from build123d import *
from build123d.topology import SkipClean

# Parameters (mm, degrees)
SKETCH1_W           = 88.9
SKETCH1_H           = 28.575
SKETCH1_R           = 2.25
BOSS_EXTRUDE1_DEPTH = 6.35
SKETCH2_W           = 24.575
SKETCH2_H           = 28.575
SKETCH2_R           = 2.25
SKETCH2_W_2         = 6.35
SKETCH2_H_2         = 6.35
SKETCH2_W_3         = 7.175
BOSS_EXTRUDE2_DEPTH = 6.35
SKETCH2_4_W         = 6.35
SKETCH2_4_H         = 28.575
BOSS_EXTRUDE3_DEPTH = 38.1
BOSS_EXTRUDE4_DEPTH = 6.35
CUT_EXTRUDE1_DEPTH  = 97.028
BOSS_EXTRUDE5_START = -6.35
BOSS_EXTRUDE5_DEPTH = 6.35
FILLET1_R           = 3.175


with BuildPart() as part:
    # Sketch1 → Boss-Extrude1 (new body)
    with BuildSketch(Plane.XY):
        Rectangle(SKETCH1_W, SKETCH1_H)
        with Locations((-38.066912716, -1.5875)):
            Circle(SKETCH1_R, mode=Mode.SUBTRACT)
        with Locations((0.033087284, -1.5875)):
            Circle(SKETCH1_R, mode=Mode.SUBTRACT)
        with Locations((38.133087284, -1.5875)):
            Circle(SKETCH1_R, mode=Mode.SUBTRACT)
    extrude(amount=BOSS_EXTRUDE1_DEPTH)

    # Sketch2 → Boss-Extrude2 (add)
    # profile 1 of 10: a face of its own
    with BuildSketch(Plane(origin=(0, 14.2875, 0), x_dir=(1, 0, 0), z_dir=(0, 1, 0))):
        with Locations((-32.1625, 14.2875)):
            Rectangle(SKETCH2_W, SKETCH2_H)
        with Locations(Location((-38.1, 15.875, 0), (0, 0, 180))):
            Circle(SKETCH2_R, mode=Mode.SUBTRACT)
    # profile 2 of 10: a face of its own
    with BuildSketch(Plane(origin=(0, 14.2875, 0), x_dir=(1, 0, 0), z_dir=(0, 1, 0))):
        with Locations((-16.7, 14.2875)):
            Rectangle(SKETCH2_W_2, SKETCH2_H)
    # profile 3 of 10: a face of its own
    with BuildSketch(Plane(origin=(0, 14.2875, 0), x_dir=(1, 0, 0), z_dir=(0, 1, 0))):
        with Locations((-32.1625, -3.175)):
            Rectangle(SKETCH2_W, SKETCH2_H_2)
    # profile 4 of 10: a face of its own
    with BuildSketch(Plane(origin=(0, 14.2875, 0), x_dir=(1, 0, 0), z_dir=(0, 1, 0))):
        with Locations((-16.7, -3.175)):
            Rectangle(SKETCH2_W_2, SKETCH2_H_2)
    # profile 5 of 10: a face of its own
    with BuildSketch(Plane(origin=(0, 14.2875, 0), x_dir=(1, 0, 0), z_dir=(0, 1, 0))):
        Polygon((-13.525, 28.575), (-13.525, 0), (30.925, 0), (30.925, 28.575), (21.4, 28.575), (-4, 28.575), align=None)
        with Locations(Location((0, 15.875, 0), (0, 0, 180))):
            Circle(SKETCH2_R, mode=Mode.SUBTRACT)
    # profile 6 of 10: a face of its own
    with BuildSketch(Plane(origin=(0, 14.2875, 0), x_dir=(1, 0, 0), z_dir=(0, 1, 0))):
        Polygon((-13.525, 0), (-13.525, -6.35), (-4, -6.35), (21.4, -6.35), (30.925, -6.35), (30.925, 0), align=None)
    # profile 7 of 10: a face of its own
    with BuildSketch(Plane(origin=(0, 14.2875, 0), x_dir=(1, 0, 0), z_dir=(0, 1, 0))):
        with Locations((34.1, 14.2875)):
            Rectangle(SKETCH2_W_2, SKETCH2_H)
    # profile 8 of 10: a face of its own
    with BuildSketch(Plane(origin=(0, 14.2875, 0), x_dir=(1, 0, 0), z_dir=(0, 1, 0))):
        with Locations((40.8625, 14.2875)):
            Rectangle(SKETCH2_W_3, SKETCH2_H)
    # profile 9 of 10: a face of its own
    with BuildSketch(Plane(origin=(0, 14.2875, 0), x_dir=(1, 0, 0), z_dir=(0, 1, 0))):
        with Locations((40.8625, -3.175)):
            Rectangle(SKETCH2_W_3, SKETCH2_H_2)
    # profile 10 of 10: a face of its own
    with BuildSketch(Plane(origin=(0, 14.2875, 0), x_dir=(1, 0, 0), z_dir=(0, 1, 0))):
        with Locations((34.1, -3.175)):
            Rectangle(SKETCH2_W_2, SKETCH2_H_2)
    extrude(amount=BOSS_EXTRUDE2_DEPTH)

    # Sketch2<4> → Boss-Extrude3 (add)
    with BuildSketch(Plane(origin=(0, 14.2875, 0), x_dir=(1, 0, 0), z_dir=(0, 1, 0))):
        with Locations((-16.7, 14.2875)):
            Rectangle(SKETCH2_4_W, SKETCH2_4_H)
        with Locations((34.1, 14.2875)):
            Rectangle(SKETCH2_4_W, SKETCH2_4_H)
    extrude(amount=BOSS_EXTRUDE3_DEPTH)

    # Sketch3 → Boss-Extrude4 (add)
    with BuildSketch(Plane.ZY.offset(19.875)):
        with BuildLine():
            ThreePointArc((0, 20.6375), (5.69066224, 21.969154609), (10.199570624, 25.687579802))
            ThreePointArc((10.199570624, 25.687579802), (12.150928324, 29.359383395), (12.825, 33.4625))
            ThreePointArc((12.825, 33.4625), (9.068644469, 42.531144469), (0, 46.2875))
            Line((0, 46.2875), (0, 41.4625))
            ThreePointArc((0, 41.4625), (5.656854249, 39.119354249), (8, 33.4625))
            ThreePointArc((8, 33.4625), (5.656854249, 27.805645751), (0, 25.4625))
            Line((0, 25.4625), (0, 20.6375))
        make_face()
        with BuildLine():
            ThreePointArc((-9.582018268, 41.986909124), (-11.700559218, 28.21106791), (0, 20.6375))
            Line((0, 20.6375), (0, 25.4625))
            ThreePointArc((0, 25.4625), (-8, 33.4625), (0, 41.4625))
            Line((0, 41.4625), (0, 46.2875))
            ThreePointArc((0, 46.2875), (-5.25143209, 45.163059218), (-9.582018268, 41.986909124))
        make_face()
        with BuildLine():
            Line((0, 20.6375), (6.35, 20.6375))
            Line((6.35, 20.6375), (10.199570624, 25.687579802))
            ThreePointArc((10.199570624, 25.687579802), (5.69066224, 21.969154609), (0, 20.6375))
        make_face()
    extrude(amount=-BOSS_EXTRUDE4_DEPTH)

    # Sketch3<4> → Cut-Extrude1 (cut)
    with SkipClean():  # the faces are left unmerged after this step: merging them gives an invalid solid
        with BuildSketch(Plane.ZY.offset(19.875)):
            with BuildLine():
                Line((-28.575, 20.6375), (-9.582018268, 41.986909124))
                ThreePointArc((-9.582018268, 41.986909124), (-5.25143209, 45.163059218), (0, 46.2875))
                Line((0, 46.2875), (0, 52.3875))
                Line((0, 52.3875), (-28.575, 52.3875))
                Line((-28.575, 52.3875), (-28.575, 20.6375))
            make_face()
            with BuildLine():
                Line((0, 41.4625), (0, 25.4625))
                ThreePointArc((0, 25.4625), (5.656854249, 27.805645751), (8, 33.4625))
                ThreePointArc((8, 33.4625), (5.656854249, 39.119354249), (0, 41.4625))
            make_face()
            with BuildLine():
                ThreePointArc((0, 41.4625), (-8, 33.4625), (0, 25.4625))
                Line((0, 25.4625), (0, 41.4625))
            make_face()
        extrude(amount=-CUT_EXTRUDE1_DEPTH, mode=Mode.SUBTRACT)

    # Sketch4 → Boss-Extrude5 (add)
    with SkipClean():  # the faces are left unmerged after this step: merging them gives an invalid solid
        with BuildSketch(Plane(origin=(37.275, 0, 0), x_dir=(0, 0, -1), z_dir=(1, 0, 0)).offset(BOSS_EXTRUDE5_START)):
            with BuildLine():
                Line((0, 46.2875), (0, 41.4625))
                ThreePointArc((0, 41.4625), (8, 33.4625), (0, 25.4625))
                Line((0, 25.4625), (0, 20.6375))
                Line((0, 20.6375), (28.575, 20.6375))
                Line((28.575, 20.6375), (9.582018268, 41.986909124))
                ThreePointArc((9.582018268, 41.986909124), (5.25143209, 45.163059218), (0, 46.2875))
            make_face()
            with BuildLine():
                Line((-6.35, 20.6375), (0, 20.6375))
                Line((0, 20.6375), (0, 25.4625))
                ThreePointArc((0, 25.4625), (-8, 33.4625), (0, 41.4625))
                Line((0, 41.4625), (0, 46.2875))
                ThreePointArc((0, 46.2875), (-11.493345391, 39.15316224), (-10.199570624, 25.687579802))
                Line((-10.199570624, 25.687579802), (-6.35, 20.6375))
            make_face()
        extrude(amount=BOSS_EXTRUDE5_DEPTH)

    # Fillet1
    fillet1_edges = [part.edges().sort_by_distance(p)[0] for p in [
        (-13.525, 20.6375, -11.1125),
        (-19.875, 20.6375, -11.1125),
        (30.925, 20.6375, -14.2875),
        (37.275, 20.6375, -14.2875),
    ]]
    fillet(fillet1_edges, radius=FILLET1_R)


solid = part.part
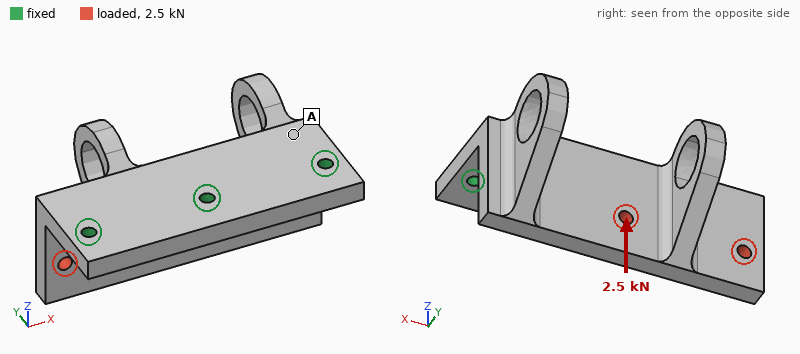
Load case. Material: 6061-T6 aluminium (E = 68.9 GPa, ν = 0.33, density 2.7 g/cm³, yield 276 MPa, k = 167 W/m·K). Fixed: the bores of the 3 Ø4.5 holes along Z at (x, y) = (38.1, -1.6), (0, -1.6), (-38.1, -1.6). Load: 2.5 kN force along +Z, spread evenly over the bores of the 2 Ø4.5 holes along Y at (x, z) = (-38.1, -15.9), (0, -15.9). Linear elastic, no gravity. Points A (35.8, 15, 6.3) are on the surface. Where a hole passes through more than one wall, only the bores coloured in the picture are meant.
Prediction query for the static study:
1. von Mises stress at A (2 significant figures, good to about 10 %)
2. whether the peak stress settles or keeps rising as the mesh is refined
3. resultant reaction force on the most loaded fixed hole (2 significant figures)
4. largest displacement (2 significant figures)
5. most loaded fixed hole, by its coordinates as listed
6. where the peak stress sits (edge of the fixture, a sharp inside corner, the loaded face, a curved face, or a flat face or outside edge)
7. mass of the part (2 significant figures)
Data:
20 MPa
keeps rising
1.4 kN
0.21 mm
(-38.1, -1.6)
edge of the fixture
110 g
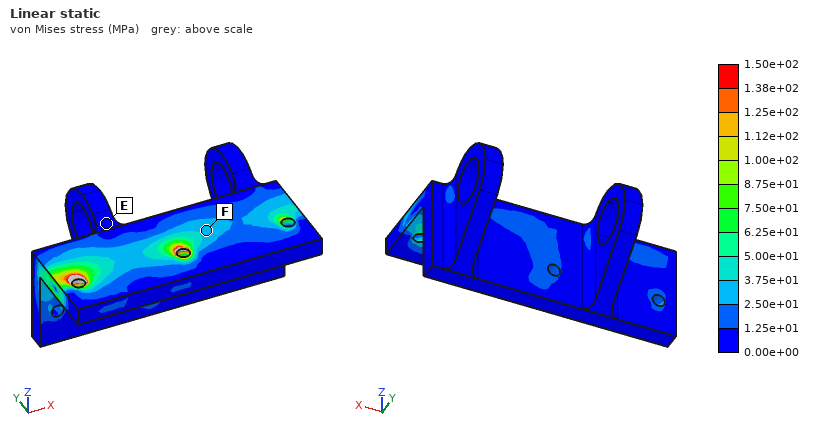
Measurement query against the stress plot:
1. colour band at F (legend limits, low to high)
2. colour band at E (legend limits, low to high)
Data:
2.50e+01 to 3.75e+01 MPa
0.00e+00 to 1.25e+01 MPa
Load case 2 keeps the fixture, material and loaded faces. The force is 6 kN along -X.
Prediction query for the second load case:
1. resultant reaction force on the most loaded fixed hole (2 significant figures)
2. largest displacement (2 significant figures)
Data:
2.7 kN
0.15 mm
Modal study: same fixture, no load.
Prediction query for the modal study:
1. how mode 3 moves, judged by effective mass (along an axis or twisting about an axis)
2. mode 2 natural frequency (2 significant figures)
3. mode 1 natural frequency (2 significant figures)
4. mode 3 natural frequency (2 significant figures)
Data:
along X
3300 Hz
2000 Hz
6600 Hz
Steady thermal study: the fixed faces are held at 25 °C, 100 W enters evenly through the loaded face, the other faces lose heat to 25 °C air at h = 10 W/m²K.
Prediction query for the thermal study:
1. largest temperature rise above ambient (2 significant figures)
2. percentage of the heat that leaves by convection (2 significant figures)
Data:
68 K
3.7 %
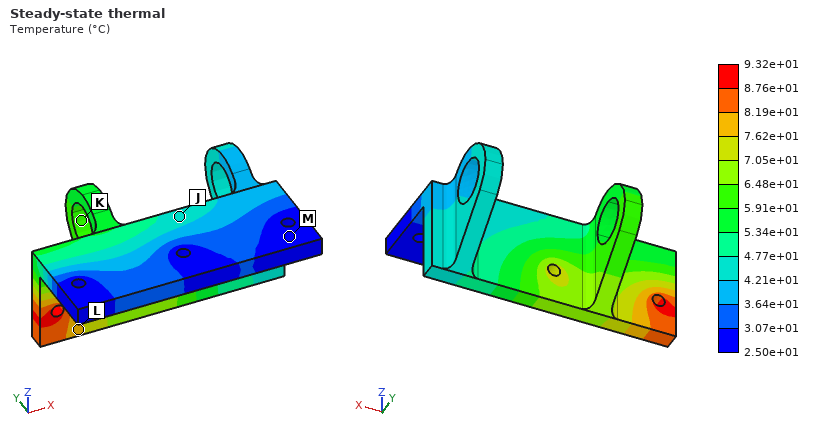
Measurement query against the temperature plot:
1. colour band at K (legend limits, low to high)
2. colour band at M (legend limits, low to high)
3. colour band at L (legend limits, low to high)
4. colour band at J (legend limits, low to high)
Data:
5.91e+01 to 6.48e+01 °C
2.50e+01 to 3.07e+01 °C
7.62e+01 to 8.19e+01 °C
4.21e+01 to 4.77e+01 °C
